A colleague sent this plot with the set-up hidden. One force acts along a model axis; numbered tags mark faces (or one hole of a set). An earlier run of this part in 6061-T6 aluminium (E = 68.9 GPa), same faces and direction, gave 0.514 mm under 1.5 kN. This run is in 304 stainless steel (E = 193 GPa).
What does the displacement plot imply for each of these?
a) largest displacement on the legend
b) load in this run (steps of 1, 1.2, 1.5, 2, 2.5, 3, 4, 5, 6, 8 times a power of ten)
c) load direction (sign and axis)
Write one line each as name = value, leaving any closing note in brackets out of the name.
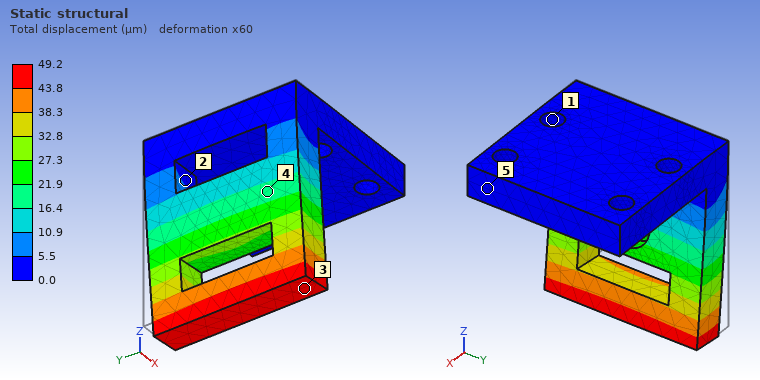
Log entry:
largest displacement on the legend = 49.2 µm
load in this run = 400 N
load direction = +X
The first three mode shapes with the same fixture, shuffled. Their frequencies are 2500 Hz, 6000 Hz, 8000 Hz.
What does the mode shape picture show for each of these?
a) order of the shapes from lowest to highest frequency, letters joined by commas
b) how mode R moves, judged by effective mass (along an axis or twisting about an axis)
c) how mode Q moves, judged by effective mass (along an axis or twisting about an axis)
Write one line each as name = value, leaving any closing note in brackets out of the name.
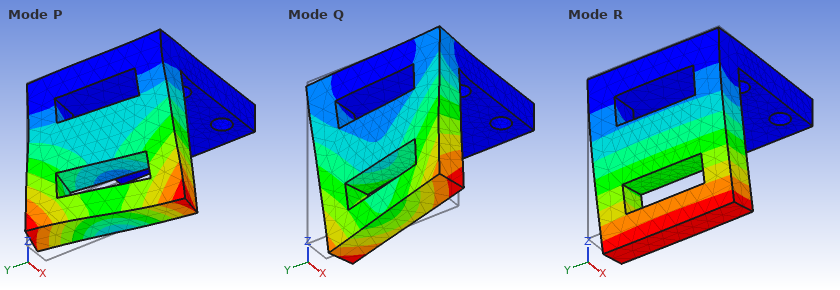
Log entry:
order of the shapes from lowest to highest frequency, letters joined by commas = R, Q, P
how mode R moves, judged by effective mass = along X
how mode Q moves, judged by effective mass = along Y
